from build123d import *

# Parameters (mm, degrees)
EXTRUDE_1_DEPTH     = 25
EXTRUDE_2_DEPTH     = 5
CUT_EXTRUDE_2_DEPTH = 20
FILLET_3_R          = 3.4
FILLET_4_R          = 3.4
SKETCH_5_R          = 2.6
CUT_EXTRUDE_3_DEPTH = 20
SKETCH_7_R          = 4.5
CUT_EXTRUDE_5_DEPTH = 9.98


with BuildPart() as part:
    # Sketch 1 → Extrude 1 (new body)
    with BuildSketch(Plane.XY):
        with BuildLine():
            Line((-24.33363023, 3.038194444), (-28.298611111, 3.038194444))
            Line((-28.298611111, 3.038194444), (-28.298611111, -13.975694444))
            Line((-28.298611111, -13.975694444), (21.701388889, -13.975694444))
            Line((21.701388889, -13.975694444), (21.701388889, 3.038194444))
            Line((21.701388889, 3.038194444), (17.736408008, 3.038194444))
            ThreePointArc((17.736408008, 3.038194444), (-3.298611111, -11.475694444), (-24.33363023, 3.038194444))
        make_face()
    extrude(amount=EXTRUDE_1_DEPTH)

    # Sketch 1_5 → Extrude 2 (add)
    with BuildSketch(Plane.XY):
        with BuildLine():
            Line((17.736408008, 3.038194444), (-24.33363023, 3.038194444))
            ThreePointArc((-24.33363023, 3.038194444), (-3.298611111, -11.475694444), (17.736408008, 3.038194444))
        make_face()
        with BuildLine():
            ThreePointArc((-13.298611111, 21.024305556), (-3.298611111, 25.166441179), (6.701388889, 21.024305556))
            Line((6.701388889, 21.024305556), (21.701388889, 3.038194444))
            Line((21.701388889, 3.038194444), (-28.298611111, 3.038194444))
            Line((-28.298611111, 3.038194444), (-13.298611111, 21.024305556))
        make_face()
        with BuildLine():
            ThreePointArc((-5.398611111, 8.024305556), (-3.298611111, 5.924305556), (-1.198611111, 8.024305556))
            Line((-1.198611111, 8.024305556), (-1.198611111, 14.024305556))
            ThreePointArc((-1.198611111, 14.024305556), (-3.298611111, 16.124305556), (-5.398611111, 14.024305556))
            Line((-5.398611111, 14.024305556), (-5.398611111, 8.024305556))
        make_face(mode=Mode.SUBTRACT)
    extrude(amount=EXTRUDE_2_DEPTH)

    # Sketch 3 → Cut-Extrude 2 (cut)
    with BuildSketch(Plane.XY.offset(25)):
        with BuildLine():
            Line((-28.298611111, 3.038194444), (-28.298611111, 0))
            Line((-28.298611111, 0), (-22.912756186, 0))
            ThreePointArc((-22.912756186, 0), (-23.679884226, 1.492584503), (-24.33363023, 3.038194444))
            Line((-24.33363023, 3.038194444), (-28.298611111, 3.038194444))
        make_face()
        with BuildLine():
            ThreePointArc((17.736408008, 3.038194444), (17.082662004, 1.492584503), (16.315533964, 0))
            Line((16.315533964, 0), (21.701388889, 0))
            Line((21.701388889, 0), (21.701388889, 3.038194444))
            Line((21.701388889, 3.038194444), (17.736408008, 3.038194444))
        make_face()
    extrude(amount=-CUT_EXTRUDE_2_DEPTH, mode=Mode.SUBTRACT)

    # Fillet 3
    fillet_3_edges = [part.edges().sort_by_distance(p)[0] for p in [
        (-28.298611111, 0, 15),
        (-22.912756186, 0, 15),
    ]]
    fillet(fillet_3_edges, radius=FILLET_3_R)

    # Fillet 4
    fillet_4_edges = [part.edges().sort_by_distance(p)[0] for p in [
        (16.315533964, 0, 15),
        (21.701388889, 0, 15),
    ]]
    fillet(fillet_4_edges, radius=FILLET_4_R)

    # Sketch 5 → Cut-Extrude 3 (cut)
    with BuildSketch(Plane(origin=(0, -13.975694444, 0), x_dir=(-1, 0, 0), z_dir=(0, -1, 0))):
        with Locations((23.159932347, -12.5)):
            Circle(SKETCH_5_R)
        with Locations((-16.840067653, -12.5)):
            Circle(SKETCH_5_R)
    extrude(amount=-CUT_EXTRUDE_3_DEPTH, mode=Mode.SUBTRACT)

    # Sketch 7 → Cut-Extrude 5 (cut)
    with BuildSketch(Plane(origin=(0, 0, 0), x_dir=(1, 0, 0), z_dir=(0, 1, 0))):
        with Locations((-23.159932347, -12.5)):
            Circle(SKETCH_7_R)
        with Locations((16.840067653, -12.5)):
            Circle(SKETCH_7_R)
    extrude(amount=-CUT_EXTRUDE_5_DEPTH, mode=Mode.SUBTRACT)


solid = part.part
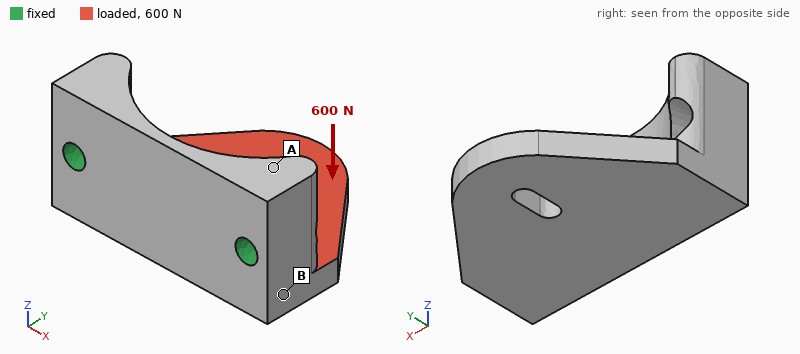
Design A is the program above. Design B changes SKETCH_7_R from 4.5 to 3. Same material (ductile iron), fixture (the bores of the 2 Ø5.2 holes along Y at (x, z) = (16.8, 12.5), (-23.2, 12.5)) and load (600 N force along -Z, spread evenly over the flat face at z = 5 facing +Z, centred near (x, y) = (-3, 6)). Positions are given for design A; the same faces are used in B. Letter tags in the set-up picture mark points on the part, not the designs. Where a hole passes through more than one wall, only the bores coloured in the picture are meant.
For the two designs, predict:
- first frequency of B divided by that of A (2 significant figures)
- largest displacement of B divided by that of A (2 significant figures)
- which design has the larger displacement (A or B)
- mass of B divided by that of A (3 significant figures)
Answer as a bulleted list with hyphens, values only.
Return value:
- 1.1
- 0.80
- A
- 1.04
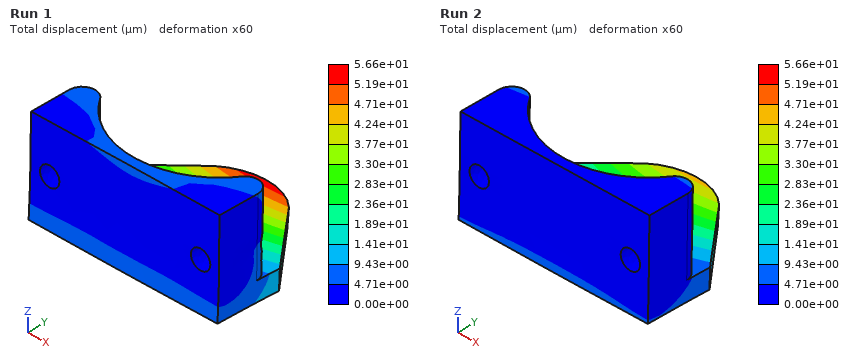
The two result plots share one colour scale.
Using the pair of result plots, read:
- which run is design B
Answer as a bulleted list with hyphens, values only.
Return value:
- Run 2
